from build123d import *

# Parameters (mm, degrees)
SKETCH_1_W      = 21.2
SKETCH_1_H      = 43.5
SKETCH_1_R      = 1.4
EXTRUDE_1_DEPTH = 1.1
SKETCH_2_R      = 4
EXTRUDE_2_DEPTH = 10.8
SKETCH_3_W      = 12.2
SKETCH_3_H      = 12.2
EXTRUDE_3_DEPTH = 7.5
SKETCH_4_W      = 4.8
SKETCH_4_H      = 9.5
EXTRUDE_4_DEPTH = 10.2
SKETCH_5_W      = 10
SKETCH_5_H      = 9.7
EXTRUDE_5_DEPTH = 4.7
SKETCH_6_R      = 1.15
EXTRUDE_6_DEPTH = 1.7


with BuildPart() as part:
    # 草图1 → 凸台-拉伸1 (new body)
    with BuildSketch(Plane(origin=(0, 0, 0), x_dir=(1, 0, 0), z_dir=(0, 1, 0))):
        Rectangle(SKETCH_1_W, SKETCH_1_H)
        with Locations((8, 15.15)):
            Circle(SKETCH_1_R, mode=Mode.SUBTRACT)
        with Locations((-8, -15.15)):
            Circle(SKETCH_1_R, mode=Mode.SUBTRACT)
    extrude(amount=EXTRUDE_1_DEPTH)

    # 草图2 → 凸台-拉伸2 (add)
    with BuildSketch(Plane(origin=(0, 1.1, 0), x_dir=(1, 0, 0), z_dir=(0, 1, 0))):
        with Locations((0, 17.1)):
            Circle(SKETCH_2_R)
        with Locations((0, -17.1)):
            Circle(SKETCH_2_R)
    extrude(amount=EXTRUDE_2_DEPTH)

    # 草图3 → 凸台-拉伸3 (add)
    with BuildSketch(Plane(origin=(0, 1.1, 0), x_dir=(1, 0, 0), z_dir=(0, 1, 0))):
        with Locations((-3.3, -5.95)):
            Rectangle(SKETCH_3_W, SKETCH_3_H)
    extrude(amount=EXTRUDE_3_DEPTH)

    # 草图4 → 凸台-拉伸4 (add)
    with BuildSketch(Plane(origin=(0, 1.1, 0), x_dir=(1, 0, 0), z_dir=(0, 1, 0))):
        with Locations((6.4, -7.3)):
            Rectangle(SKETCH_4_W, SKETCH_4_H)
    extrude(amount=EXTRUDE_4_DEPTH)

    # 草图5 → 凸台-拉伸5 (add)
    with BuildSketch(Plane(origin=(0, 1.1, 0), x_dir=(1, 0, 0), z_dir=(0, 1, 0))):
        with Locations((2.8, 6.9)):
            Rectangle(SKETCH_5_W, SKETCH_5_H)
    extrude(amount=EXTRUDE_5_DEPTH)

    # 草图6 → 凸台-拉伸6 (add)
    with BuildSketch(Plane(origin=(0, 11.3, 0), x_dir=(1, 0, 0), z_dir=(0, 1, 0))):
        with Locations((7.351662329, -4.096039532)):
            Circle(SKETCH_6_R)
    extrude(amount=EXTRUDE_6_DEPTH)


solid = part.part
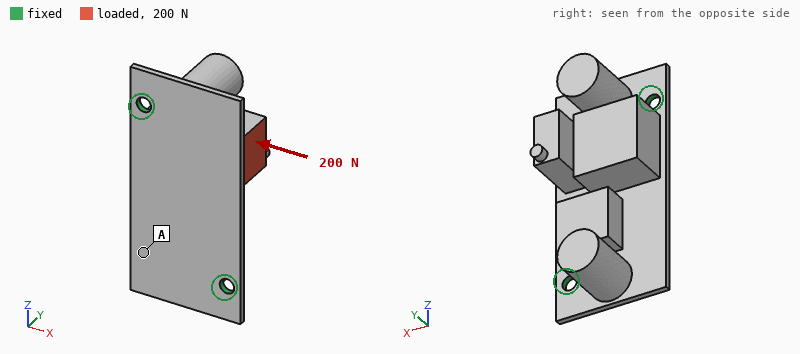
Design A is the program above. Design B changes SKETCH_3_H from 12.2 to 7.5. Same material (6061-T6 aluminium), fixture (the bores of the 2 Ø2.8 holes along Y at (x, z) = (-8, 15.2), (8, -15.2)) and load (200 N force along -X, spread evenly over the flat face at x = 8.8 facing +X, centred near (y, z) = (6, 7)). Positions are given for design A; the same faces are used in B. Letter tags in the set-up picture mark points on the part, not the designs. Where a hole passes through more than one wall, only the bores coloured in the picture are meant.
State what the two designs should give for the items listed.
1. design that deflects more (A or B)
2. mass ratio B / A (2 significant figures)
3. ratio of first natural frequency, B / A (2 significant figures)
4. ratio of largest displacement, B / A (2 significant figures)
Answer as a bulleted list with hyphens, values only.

- B
- 0.90
- 0.91
- 1.1
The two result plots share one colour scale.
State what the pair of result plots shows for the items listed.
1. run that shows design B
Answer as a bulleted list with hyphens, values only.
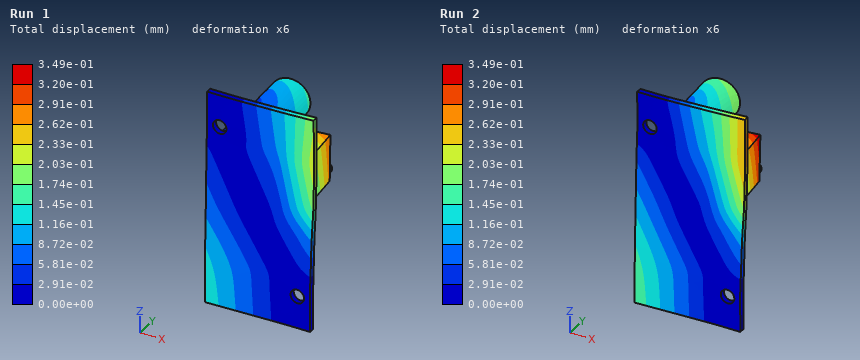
- Run 2
